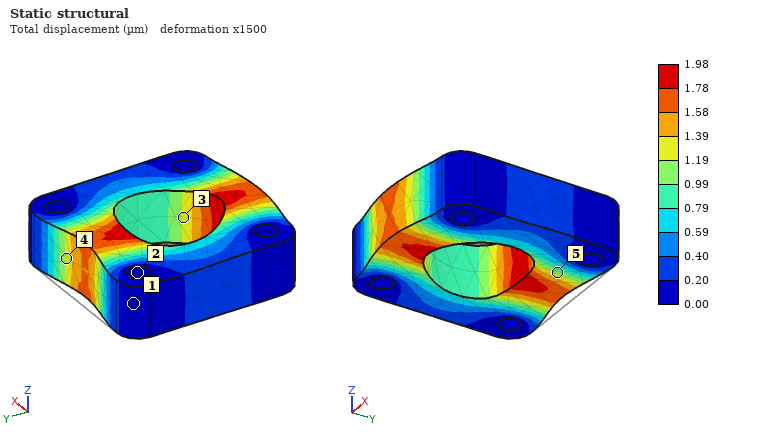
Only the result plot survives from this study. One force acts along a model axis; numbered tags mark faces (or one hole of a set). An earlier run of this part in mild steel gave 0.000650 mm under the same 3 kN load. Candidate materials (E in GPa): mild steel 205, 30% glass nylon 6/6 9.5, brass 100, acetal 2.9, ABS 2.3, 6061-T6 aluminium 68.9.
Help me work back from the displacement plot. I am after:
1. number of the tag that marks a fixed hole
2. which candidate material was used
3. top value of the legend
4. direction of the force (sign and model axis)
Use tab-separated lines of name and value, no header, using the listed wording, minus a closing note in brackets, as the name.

number of the tag that marks a fixed hole	2
which candidate material was used	6061-T6 aluminium
top value of the legend	1.98 µm
direction of the force	-Y
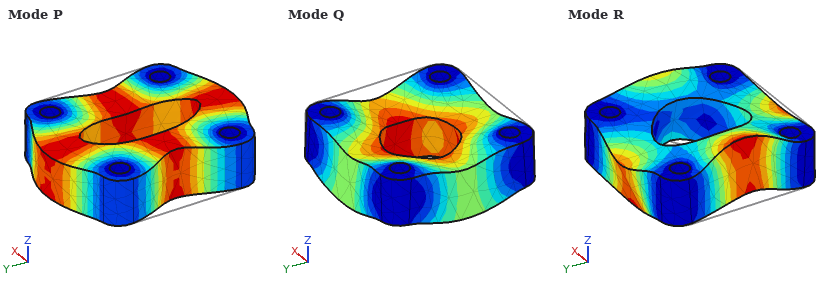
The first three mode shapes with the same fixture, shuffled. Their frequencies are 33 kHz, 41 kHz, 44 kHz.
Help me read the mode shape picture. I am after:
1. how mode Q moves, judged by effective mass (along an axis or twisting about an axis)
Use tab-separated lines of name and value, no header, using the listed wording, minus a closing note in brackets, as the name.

how mode Q moves, judged by effective mass	along Z
